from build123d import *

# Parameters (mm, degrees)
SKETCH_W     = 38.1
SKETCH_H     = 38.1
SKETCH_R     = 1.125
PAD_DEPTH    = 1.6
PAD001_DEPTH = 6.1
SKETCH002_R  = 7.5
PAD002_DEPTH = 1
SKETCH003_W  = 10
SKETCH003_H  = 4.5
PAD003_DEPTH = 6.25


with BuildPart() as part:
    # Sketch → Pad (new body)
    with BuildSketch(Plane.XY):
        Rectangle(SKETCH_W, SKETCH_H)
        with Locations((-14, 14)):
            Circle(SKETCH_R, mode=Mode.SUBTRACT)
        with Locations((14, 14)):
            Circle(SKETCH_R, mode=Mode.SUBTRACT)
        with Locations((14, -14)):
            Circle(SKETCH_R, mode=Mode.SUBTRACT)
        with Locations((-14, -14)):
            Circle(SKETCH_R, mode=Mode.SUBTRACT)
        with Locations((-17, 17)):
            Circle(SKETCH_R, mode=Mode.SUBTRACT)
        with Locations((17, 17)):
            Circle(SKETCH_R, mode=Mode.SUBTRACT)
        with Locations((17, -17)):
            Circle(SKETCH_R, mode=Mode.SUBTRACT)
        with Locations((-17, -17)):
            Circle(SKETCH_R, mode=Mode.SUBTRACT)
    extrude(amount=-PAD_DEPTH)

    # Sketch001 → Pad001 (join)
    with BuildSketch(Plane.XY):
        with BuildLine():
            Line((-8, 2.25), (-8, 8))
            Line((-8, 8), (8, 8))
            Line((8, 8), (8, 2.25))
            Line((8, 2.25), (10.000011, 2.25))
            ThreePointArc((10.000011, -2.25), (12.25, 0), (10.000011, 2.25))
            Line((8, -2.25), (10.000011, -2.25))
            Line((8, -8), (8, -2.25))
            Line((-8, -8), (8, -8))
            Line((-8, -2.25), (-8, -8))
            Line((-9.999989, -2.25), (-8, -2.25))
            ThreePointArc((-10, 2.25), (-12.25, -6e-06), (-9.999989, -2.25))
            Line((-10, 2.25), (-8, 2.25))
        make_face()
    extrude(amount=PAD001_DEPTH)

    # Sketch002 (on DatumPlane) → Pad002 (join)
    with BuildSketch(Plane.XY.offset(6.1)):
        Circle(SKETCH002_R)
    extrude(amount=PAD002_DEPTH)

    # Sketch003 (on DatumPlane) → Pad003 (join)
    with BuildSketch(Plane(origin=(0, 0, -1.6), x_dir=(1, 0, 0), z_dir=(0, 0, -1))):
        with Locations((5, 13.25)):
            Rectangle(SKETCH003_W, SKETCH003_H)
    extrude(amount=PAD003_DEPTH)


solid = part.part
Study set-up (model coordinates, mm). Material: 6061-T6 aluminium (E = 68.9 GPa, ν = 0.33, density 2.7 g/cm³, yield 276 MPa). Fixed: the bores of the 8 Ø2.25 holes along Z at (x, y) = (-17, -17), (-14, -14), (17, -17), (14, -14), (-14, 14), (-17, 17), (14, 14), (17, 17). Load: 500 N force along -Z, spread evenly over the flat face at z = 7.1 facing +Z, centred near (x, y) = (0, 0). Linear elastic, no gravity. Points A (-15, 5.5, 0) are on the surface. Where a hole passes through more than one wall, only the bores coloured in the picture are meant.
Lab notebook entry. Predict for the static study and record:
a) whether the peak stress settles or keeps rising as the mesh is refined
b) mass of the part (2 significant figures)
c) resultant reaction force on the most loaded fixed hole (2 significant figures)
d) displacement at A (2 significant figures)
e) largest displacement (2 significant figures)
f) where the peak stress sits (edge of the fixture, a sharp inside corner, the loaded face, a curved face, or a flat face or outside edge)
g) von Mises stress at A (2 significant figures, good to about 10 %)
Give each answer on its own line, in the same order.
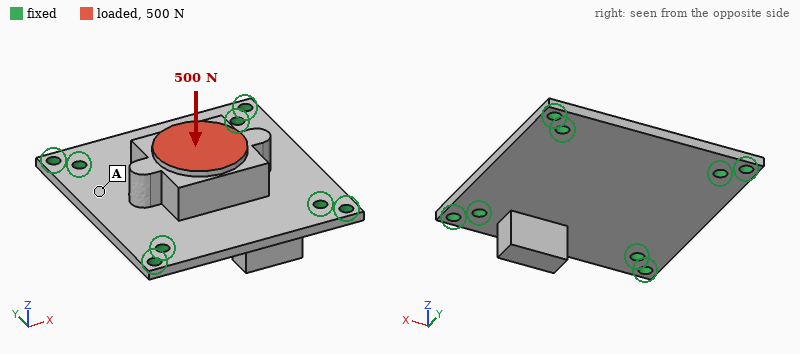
keeps rising
12 g
170 N
23 µm
39 µm
edge of the fixture
21 MPa
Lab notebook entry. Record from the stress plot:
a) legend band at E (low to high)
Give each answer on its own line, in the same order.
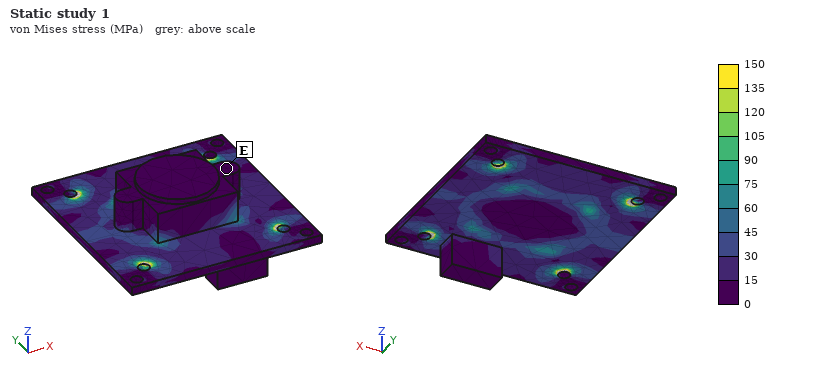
0 to 15 MPa
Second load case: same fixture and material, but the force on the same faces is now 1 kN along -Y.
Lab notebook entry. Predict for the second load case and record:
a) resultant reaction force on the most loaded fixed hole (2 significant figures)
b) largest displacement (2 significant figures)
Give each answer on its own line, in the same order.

310 N
56 µm
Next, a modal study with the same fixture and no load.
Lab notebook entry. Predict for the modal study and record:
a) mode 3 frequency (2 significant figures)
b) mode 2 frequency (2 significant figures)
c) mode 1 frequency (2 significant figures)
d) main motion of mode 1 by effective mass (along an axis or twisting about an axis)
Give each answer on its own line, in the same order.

10 kHz
9700 Hz
6400 Hz
along Z
